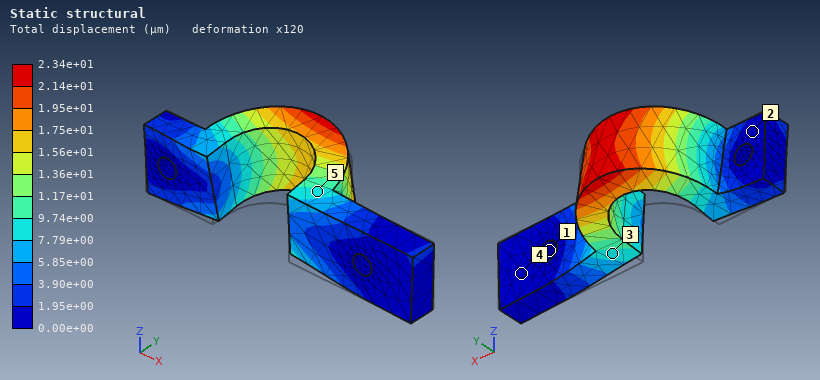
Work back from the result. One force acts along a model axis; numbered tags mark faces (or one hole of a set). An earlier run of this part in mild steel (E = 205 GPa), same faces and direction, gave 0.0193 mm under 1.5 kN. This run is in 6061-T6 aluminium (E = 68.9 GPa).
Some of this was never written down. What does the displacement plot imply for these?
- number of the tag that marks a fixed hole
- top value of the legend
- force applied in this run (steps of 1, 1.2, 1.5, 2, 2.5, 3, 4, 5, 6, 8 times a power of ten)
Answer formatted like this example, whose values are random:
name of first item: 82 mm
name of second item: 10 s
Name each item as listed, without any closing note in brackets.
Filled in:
number of the tag that marks a fixed hole: 1
top value of the legend: 2.34e+01 µm
force applied in this run: 600 N
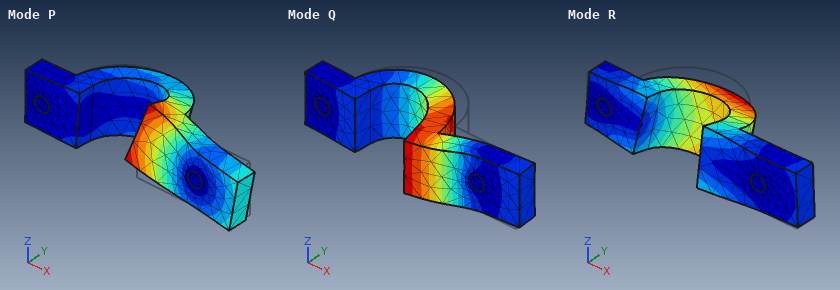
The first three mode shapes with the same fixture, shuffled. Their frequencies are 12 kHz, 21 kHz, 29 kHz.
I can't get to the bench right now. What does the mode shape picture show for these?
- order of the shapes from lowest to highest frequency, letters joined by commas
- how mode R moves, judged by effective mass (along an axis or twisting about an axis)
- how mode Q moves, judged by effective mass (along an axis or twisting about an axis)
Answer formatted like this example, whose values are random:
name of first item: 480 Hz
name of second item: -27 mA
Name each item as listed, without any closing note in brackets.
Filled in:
order of the shapes from lowest to highest frequency, letters joined by commas: R, Q, P
how mode R moves, judged by effective mass: along Z
how mode Q moves, judged by effective mass: along Y
